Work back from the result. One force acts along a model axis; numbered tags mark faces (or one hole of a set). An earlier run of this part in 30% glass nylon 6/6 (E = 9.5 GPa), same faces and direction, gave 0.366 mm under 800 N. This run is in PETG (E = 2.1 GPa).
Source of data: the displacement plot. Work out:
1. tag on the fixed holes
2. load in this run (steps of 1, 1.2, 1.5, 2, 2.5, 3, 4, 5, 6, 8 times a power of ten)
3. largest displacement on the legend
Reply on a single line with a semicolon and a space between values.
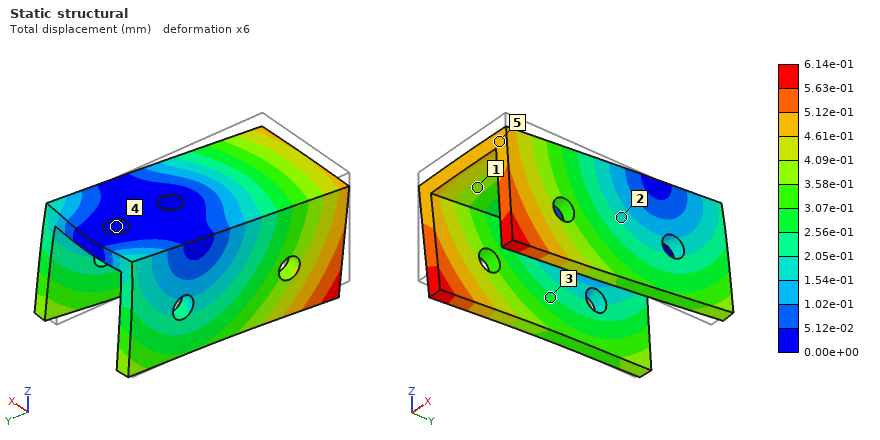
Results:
4; 300 N; 6.14e-01 mm
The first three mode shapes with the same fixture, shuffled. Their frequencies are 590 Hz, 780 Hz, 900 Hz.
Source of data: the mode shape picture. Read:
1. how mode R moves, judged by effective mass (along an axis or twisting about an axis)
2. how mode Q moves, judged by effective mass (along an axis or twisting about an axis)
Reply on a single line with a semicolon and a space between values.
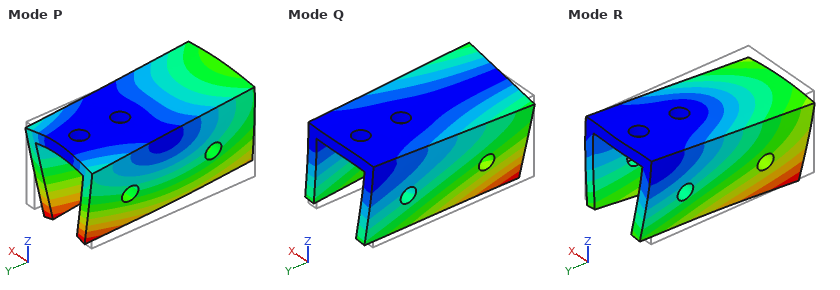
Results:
along Z; along X
